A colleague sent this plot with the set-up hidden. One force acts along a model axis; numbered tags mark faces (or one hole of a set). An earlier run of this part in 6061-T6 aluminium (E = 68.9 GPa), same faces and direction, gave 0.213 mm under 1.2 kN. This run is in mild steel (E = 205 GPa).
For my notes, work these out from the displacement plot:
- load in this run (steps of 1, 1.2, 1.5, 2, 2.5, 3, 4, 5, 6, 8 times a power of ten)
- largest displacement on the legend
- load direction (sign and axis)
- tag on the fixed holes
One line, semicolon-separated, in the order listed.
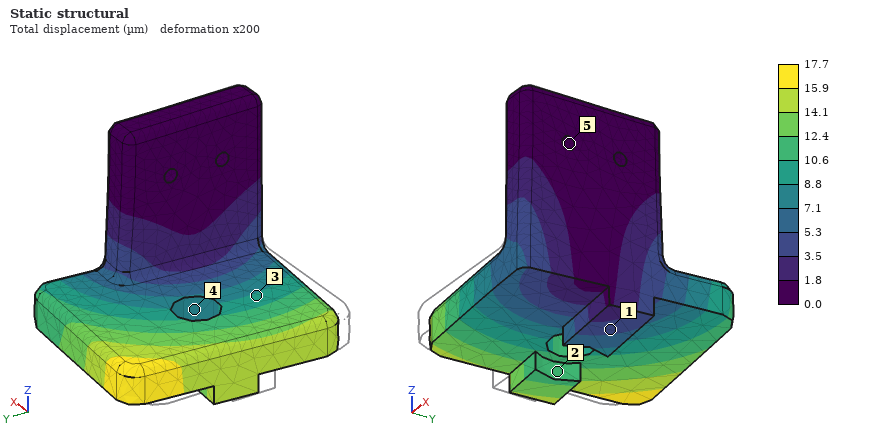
300 N; 17.7 µm; +Y; 5
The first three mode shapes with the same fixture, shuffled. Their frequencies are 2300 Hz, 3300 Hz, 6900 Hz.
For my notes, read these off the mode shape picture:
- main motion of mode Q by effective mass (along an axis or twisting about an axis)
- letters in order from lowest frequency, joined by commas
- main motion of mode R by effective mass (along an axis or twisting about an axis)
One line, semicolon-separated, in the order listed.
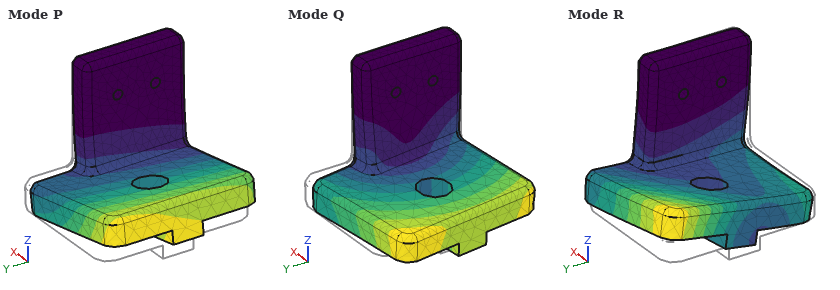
along Y; P, Q, R; along X
